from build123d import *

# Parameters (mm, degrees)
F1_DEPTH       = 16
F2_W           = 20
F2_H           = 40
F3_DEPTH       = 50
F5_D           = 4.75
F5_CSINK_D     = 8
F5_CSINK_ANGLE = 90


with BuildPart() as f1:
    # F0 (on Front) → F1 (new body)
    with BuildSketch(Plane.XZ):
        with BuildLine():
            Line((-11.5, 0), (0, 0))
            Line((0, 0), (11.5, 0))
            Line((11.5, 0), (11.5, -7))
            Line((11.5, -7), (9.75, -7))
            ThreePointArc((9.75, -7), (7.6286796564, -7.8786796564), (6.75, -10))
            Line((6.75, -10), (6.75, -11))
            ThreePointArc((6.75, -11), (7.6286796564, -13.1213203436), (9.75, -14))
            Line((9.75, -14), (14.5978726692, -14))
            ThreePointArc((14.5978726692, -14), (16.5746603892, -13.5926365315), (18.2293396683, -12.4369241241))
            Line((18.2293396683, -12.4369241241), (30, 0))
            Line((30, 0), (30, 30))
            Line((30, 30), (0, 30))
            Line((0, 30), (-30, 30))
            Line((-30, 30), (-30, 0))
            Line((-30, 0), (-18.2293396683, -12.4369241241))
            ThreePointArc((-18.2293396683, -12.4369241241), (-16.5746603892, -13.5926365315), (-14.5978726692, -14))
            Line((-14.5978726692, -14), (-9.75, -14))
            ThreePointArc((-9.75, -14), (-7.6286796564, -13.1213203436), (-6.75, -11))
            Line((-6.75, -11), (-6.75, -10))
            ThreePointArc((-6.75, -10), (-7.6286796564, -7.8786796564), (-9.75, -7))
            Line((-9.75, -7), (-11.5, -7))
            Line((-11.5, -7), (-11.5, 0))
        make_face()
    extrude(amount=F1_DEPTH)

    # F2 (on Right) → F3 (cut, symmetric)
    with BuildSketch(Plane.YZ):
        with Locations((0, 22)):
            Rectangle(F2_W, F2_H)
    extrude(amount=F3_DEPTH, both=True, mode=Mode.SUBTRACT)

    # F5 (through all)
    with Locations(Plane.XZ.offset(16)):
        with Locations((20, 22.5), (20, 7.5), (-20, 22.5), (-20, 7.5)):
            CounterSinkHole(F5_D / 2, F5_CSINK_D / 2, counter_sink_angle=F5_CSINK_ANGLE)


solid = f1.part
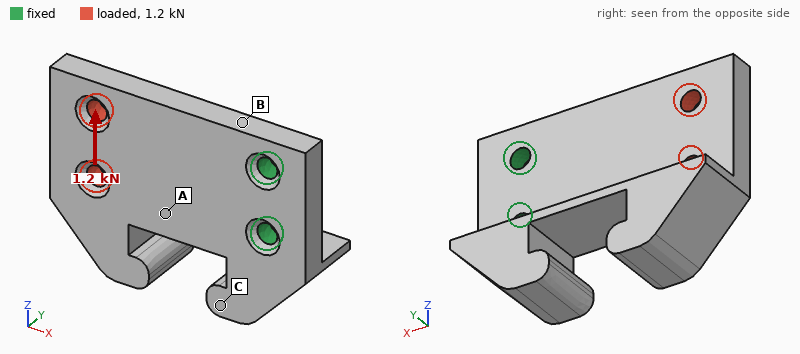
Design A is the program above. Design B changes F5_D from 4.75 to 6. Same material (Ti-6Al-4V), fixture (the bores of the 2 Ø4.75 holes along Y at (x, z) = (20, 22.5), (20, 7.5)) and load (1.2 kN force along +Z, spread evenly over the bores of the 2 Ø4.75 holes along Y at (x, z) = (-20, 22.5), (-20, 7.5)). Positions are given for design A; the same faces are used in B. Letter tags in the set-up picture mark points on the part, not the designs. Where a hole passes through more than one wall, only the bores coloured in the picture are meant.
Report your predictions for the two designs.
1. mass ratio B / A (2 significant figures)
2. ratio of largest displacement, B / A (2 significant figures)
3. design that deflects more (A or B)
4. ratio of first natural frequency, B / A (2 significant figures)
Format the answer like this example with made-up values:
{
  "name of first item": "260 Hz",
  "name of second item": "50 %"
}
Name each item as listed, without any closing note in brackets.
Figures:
{
  "mass ratio B / A": "0.99",
  "ratio of largest displacement, B / A": "0.85",
  "design that deflects more": "A",
  "ratio of first natural frequency, B / A": "1.1"
}
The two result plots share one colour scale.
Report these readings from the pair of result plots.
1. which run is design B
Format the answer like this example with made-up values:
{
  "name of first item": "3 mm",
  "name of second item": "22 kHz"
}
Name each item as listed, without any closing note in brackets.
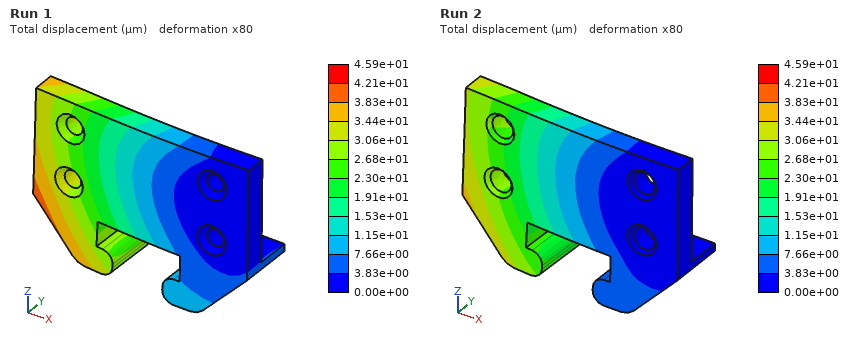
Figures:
{
  "which run is design B": "Run 2"
}
